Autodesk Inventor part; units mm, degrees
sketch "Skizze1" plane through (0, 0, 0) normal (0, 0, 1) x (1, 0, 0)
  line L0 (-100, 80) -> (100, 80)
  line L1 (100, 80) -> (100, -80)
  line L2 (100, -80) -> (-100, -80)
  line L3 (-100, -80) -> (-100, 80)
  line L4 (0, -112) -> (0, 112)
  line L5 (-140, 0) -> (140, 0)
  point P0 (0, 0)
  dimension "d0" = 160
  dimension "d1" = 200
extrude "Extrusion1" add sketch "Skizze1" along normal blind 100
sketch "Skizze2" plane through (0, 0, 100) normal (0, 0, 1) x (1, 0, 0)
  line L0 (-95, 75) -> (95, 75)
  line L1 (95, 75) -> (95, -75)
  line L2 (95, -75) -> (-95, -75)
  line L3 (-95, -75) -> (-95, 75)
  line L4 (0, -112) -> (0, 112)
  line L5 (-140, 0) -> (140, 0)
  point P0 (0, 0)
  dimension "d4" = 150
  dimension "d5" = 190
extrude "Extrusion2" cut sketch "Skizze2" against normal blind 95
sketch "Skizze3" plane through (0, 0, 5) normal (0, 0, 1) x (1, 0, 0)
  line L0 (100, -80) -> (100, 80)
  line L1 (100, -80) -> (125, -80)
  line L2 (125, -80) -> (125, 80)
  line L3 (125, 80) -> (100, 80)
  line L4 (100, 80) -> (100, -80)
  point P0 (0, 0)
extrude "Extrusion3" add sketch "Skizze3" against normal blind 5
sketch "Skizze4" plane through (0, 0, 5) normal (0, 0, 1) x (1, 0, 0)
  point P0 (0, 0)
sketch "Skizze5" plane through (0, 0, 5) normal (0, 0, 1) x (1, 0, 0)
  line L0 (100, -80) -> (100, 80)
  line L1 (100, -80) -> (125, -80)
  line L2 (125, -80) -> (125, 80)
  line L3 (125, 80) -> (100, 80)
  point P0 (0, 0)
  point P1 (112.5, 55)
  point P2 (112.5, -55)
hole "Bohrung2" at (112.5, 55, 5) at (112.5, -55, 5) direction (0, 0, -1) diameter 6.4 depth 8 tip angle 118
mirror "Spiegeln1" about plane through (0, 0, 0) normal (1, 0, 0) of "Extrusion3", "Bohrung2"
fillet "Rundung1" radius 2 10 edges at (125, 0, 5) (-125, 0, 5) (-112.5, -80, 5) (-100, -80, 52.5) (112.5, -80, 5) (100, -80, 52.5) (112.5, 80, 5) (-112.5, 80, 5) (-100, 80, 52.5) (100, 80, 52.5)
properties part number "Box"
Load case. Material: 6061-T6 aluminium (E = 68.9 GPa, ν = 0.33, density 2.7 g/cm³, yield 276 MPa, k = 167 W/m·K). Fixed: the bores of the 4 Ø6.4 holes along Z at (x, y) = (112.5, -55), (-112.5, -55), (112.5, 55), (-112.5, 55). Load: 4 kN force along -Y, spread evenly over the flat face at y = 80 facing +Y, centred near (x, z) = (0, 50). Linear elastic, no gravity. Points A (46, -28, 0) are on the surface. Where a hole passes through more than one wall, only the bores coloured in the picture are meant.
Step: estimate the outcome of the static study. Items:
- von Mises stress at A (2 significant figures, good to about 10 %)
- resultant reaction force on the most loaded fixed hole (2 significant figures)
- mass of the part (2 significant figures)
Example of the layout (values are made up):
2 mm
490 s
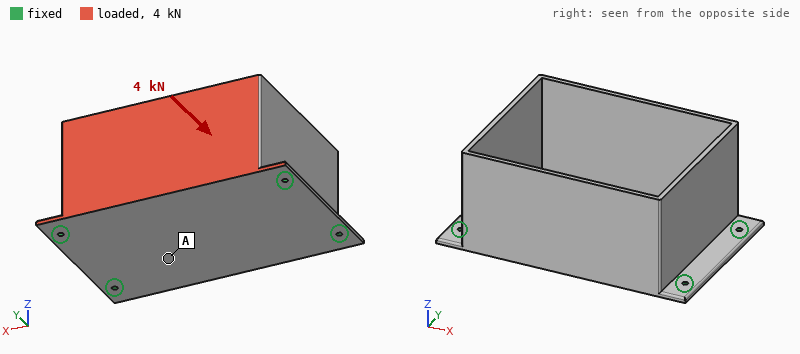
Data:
8.6 MPa
1.5 kN
1.4 kg
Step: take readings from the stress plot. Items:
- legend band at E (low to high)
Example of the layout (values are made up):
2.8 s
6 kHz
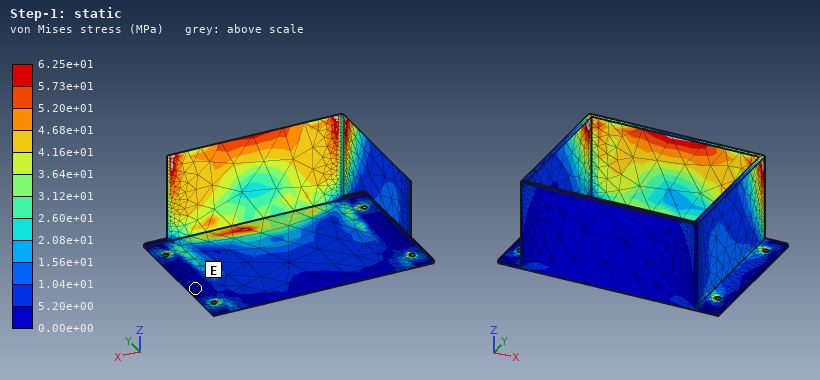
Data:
0.00e+00 to 5.20e+00 MPa
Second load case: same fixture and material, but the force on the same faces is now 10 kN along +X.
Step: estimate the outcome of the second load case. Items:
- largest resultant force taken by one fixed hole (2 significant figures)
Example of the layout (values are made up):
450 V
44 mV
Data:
5.0 kN
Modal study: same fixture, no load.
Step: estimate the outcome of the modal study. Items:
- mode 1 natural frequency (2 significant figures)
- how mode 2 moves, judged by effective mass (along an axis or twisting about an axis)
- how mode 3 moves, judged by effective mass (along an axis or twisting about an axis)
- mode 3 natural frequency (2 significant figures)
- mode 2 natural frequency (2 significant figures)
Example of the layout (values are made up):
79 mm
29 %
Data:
690 Hz
along Y
along X
1000 Hz
750 Hz
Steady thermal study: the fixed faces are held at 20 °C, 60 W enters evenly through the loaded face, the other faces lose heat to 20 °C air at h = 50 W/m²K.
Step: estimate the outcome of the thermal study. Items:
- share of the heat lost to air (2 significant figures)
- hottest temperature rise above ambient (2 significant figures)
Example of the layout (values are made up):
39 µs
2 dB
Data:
65 %
17 K
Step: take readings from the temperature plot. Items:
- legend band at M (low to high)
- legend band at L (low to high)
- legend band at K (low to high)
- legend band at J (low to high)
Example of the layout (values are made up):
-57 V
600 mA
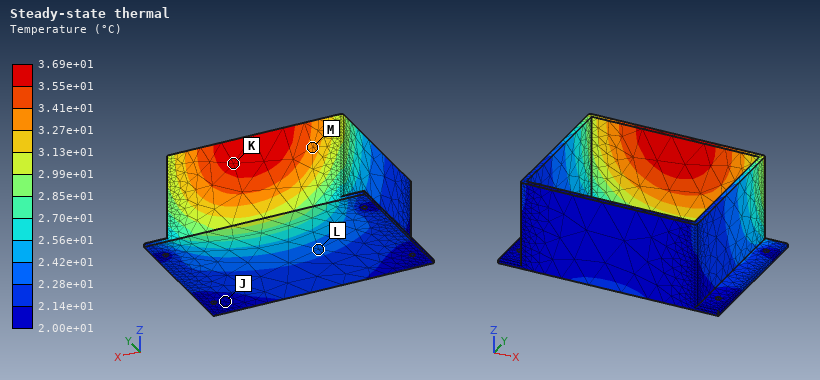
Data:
3.27e+01 to 3.41e+01 °C
2.28e+01 to 2.42e+01 °C
3.55e+01 to 3.69e+01 °C
2.00e+01 to 2.14e+01 °C
